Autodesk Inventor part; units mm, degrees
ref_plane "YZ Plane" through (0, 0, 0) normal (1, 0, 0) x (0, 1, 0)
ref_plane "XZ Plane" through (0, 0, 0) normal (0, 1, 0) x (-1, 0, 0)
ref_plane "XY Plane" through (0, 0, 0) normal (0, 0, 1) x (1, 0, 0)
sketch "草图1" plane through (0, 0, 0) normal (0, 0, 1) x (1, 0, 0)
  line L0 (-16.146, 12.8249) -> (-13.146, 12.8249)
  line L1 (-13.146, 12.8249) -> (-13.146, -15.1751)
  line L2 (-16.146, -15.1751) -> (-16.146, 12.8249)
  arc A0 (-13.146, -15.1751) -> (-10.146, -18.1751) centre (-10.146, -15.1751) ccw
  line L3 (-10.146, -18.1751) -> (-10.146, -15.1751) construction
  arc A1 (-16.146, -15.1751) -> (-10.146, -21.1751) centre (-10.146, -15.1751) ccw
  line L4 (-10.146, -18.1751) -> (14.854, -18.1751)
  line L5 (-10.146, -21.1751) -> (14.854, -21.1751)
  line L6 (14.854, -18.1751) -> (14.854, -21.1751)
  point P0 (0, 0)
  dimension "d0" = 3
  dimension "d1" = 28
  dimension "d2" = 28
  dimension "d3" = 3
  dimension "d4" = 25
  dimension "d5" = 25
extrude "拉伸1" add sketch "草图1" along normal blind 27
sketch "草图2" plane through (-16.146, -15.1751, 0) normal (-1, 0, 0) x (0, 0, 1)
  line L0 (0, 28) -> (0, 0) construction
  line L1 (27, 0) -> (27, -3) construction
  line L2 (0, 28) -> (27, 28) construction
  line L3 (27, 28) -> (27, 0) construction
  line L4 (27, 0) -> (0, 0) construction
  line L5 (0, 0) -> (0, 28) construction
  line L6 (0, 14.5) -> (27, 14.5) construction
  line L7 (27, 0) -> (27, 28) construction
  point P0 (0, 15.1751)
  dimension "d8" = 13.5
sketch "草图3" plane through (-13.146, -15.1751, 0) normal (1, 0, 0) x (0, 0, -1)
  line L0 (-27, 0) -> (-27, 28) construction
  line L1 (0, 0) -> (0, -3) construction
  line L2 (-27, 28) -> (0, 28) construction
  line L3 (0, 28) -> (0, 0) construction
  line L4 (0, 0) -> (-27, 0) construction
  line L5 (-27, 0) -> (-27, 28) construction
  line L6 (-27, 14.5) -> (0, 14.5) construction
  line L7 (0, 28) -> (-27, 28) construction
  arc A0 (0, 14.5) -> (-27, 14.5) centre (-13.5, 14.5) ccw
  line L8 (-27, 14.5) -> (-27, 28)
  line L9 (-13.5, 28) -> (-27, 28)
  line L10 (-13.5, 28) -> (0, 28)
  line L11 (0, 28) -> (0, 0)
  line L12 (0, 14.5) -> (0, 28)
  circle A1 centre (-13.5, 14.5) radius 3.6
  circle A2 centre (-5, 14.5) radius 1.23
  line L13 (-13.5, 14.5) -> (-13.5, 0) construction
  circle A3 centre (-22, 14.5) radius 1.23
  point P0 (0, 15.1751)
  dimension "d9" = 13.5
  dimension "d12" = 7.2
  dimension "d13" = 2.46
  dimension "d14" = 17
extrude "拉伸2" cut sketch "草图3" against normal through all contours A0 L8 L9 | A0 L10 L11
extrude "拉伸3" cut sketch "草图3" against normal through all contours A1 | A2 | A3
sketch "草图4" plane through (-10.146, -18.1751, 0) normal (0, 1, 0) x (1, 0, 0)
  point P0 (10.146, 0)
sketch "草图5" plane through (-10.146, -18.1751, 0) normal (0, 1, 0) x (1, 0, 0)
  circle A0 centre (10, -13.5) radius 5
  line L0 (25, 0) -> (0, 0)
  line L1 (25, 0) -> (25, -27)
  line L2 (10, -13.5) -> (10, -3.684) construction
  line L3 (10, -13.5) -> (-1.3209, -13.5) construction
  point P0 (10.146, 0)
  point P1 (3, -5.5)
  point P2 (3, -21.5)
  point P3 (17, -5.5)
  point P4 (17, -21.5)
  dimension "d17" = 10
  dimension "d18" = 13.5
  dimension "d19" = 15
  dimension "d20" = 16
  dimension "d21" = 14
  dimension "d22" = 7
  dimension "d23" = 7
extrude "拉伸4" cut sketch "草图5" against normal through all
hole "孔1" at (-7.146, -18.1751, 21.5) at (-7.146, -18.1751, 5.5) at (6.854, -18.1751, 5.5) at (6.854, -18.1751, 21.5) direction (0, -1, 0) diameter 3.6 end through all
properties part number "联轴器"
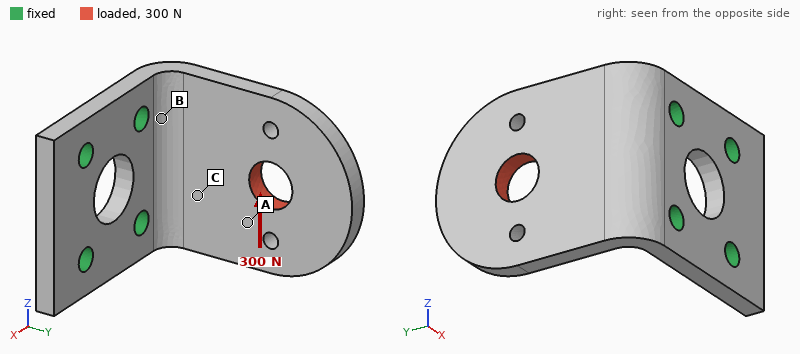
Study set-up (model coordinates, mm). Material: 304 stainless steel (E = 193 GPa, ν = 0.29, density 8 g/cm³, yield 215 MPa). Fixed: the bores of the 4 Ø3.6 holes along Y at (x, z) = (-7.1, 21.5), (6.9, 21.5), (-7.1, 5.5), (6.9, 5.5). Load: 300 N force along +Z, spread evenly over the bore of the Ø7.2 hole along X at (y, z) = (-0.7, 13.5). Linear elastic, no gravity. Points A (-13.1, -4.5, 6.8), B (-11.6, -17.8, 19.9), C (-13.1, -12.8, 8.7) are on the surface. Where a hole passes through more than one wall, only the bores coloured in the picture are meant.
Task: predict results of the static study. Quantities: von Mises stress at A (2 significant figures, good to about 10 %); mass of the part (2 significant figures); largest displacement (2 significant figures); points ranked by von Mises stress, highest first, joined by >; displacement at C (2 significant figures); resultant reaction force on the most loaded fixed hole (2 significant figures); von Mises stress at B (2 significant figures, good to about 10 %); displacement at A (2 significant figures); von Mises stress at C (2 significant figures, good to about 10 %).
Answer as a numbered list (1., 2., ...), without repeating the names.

1. 12 MPa
2. 33 g
3. 18 µm
4. B > C > A
5. 4.6 µm
6. 370 N
7. 44 MPa
8. 9.7 µm
9. 24 MPa
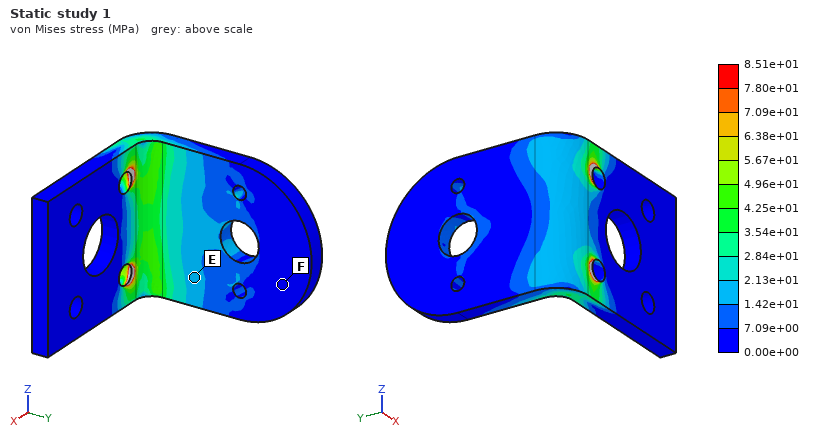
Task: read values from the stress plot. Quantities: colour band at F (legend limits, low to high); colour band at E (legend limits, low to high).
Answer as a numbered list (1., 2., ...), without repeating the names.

1. 0.00e+00 to 7.09e+00 MPa
2. 1.42e+01 to 2.13e+01 MPa
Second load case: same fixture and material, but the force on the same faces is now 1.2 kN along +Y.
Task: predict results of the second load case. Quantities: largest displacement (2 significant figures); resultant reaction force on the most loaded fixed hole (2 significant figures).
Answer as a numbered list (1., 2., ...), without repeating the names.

1. 89 µm
2. 630 N
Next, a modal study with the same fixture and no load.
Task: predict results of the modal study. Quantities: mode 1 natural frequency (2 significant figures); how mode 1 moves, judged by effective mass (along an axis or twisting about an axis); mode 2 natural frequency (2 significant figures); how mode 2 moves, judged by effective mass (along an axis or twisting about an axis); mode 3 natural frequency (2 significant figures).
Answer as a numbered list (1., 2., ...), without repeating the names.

1. 2100 Hz
2. along X
3. 5800 Hz
4. along Z
5. 8600 Hz
